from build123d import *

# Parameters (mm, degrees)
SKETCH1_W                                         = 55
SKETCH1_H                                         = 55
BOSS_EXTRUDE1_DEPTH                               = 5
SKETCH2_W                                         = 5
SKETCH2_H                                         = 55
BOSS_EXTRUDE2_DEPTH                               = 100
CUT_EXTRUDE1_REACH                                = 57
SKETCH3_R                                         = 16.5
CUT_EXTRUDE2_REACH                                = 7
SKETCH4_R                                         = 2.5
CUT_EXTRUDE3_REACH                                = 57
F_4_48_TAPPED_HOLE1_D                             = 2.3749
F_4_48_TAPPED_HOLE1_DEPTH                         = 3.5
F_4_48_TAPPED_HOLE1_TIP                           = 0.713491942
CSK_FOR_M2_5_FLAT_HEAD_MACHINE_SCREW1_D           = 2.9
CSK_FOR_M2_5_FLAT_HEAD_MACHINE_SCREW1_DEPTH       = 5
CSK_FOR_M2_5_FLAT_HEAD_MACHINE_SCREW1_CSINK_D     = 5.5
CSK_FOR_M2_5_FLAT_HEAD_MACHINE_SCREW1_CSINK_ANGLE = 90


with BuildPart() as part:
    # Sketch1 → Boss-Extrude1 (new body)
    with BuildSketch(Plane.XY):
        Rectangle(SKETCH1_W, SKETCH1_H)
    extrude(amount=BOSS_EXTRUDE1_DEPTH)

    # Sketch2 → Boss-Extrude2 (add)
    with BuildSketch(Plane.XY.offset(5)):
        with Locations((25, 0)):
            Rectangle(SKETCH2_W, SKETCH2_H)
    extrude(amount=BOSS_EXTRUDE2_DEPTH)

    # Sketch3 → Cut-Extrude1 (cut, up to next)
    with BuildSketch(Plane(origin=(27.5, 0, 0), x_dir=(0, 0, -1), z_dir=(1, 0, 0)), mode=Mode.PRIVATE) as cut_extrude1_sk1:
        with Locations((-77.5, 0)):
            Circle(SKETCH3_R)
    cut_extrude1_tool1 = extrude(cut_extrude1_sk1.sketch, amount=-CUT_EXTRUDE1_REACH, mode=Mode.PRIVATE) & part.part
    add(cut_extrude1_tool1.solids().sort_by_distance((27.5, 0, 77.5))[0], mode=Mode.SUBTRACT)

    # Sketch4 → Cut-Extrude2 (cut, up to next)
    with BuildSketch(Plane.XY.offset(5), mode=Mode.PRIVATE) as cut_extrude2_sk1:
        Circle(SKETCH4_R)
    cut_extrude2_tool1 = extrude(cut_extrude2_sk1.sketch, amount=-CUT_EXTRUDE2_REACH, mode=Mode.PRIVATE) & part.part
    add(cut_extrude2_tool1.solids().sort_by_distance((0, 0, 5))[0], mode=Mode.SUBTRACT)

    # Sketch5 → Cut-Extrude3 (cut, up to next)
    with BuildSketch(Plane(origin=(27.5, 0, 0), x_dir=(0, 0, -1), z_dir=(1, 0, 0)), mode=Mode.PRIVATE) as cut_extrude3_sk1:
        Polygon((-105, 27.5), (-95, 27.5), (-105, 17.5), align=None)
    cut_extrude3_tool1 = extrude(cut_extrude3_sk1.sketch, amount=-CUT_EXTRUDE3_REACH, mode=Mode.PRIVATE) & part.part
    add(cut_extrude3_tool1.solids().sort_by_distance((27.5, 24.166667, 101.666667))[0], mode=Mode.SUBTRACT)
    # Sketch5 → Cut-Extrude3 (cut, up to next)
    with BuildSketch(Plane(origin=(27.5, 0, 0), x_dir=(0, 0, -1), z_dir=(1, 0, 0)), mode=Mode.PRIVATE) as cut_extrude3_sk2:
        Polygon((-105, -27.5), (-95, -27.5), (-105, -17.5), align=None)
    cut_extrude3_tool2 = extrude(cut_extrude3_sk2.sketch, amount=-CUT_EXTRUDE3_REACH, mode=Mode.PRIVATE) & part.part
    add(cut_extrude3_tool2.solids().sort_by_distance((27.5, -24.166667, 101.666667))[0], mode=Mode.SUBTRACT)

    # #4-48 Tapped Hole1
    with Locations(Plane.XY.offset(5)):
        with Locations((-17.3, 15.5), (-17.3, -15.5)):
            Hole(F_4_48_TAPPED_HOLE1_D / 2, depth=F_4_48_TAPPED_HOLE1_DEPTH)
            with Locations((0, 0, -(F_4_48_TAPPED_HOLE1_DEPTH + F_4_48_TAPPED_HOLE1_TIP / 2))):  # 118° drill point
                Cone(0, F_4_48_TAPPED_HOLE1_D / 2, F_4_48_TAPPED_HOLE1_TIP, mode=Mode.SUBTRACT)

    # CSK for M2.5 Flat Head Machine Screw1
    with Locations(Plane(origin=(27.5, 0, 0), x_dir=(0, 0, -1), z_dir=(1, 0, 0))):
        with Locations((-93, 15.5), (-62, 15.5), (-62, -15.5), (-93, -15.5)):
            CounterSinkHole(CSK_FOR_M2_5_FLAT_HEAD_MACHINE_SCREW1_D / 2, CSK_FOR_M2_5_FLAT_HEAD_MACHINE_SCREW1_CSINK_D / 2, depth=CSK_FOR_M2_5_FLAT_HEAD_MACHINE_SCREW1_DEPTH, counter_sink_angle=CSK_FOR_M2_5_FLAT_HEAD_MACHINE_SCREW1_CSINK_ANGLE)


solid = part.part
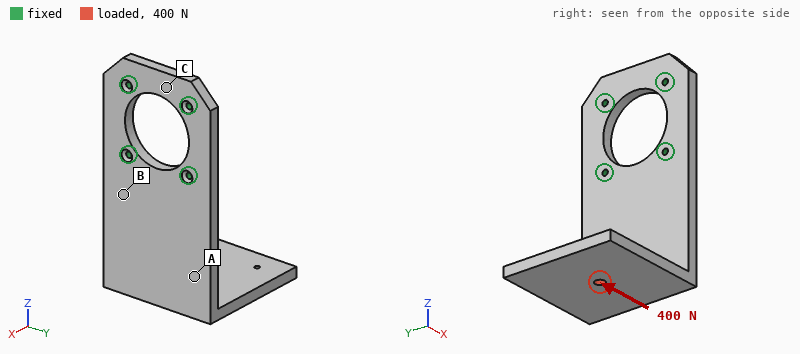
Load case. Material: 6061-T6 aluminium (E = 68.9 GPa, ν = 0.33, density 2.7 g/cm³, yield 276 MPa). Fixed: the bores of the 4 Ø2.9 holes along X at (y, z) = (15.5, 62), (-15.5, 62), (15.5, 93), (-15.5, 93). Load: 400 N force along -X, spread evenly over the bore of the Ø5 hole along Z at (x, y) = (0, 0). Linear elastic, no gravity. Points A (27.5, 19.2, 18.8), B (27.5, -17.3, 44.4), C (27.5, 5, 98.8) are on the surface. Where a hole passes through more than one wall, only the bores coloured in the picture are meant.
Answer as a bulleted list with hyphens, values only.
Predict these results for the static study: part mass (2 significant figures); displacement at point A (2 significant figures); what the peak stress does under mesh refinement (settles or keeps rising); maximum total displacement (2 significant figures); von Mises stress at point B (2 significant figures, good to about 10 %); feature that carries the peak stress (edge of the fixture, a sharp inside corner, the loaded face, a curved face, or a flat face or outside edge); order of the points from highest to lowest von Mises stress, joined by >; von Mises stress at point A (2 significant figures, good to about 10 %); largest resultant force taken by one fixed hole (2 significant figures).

- 100 g
- 0.58 mm
- keeps rising
- 1.5 mm
- 70 MPa
- edge of the fixture
- B > A > C
- 30 MPa
- 340 N
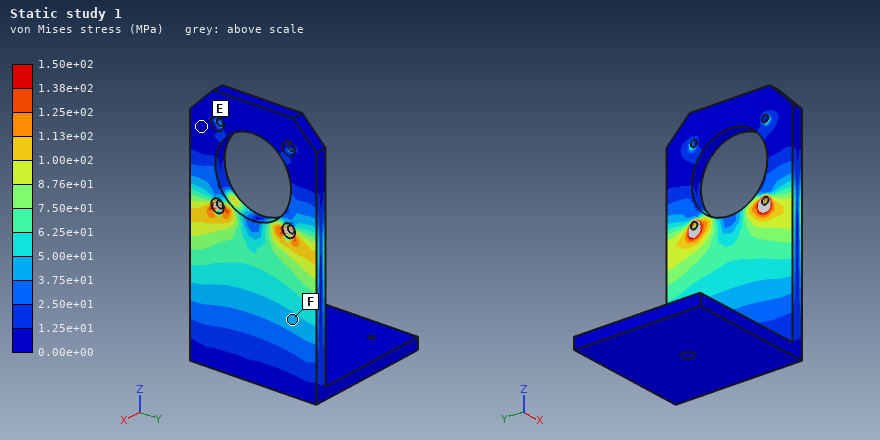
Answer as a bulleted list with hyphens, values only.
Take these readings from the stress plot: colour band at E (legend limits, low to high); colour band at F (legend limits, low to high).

- 0.00e+00 to 1.25e+01 MPa
- 3.75e+01 to 5.00e+01 MPa
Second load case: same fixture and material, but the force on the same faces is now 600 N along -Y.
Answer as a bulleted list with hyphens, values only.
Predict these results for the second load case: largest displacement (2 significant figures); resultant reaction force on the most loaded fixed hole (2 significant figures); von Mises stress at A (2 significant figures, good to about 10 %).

- 0.70 mm
- 910 N
- 43 MPa
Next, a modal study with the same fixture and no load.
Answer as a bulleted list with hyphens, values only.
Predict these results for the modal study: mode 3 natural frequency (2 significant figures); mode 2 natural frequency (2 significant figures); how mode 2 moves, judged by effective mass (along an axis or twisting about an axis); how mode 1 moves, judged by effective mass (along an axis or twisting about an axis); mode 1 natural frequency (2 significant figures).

- 1200 Hz
- 810 Hz
- along Y
- along X
- 390 Hz
